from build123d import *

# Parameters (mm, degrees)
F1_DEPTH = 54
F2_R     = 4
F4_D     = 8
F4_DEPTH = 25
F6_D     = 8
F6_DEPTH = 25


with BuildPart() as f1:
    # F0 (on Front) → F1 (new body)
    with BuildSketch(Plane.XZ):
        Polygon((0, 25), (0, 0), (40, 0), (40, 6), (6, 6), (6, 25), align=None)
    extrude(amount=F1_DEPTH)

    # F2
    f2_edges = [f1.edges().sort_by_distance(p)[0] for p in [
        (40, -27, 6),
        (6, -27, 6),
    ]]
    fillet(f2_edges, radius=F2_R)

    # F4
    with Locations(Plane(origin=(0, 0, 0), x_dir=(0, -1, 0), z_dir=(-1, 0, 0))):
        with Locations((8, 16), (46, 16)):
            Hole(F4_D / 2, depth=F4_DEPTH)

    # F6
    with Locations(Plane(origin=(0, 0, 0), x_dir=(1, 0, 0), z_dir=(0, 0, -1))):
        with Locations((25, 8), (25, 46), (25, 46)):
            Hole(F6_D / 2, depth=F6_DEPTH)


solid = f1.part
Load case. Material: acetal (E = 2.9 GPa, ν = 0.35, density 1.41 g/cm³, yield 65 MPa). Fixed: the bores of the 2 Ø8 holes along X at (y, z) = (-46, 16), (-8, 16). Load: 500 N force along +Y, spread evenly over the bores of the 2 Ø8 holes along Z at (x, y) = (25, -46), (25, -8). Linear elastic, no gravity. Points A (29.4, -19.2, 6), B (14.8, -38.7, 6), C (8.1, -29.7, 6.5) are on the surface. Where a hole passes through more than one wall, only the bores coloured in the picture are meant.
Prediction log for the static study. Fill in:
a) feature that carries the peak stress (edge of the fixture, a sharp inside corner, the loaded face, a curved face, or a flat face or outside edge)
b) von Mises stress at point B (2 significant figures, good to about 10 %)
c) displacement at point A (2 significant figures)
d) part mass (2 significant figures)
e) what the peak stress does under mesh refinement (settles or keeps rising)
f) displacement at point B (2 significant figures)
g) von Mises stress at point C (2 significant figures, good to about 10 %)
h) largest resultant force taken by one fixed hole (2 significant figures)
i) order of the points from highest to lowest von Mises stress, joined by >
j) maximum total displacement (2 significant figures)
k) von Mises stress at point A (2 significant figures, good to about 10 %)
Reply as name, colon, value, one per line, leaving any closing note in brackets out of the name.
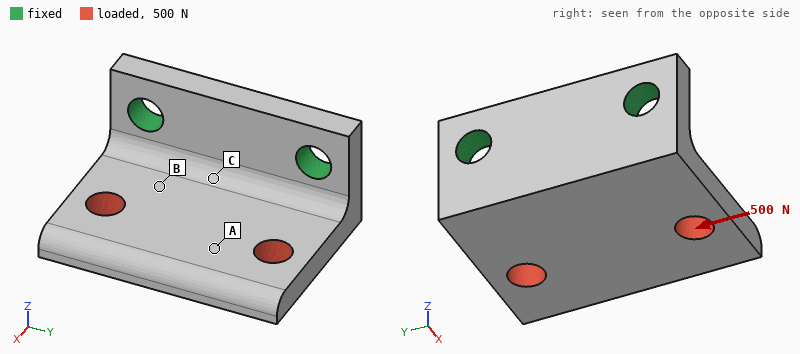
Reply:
feature that carries the peak stress: edge of the fixture
von Mises stress at point B: 6.2 MPa
displacement at point A: 0.17 mm
part mass: 25 g
what the peak stress does under mesh refinement: keeps rising
displacement at point B: 0.098 mm
von Mises stress at point C: 9.5 MPa
largest resultant force taken by one fixed hole: 390 N
order of the points from highest to lowest von Mises stress, joined by >: C > B > A
maximum total displacement: 0.28 mm
von Mises stress at point A: 2.5 MPa
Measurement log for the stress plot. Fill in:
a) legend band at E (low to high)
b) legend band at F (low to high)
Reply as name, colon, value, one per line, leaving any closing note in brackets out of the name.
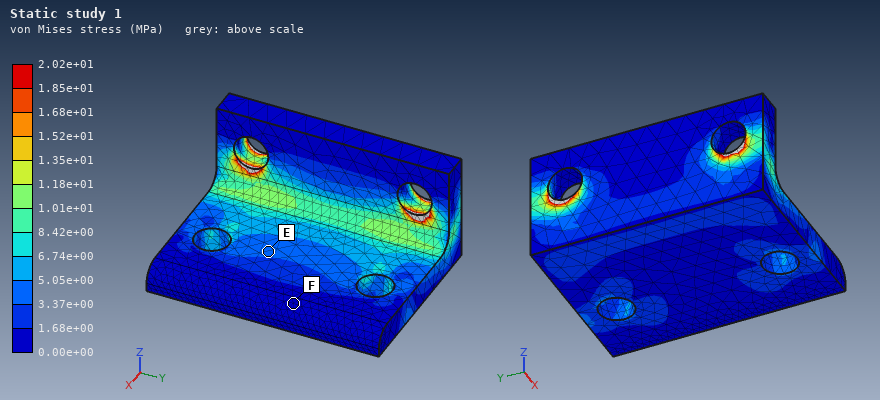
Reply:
legend band at E: 3.37e+00 to 5.05e+00 MPa
legend band at F: 0.00e+00 to 1.68e+00 MPa
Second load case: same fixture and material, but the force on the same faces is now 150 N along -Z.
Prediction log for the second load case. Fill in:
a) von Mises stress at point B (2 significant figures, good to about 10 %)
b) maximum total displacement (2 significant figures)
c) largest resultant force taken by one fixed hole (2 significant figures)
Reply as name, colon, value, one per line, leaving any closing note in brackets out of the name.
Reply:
von Mises stress at point B: 4.3 MPa
maximum total displacement: 0.66 mm
largest resultant force taken by one fixed hole: 76 N
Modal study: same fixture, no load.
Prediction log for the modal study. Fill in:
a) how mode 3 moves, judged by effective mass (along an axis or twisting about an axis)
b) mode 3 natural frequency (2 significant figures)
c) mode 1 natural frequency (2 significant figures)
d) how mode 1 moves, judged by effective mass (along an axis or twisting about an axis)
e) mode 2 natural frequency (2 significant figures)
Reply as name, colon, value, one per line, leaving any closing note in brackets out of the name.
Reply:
how mode 3 moves, judged by effective mass: along Y
mode 3 natural frequency: 2600 Hz
mode 1 natural frequency: 810 Hz
how mode 1 moves, judged by effective mass: along Z
mode 2 natural frequency: 1600 Hz
